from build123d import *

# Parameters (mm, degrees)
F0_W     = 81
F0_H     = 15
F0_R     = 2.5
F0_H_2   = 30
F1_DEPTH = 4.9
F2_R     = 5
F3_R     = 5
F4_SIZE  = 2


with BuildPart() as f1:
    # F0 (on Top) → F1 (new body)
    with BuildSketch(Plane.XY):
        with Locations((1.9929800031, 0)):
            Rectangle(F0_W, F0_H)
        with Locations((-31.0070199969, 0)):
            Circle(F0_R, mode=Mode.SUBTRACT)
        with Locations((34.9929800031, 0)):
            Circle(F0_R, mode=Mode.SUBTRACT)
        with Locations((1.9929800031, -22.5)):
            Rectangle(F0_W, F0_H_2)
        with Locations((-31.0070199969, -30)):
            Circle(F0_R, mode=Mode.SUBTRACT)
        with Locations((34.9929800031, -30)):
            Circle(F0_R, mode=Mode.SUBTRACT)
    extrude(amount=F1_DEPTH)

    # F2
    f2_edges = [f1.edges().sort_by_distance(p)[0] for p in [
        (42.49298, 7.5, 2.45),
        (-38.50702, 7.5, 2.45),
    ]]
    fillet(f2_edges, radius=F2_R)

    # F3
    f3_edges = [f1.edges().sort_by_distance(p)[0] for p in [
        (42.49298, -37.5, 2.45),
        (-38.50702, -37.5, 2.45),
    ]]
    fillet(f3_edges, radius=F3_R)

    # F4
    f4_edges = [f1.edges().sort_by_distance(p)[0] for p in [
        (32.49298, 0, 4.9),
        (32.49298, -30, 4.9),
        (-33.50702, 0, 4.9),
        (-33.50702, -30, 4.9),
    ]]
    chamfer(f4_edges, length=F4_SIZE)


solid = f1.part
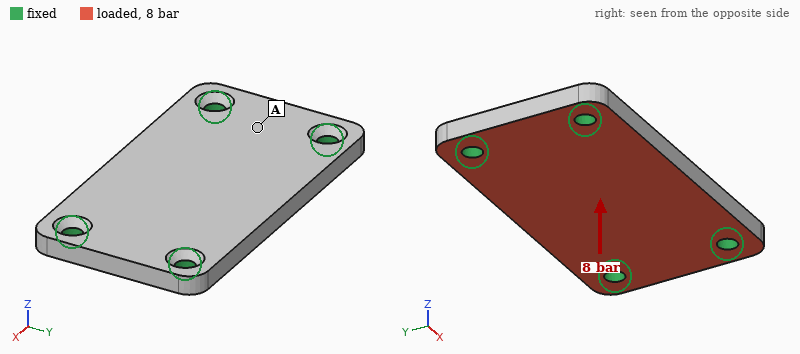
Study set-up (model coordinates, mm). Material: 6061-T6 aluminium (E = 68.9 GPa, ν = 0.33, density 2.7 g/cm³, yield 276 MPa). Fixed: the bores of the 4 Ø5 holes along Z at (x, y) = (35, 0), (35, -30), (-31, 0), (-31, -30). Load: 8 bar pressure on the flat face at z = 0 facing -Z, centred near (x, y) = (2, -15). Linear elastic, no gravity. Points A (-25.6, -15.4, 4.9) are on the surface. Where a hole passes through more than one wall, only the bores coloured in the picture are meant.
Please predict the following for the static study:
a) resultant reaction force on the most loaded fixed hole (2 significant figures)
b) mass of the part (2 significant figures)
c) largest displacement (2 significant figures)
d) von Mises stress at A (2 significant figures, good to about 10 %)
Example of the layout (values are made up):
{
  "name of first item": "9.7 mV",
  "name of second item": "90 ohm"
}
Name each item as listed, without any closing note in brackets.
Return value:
{
  "resultant reaction force on the most loaded fixed hole": "800 N",
  "mass of the part": "46 g",
  "largest displacement": "83 µm",
  "von Mises stress at A": "23 MPa"
}
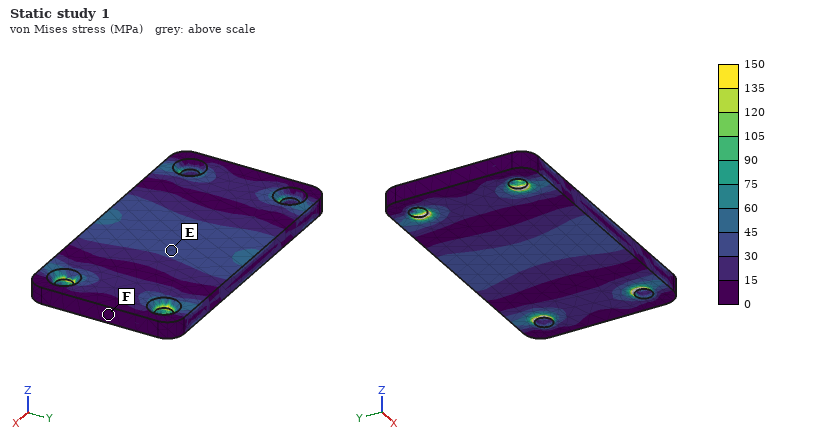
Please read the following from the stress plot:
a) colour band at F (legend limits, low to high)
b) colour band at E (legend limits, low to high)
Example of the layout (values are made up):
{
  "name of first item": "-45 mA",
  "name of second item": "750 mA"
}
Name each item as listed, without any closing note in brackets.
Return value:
{
  "colour band at F": "0 to 15 MPa",
  "colour band at E": "30 to 45 MPa"
}
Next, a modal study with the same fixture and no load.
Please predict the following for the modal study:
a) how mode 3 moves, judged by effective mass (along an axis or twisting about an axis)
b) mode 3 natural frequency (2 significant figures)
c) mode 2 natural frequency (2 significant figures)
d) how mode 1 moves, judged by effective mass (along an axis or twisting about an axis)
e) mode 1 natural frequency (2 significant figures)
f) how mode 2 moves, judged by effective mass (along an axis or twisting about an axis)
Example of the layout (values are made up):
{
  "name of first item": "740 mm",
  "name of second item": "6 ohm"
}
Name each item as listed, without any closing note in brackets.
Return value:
{
  "how mode 3 moves, judged by effective mass": "twisting about Y",
  "mode 3 natural frequency": "13 kHz",
  "mode 2 natural frequency": "7300 Hz",
  "how mode 1 moves, judged by effective mass": "along Z",
  "mode 1 natural frequency": "4900 Hz",
  "how mode 2 moves, judged by effective mass": "twisting about X"
}
